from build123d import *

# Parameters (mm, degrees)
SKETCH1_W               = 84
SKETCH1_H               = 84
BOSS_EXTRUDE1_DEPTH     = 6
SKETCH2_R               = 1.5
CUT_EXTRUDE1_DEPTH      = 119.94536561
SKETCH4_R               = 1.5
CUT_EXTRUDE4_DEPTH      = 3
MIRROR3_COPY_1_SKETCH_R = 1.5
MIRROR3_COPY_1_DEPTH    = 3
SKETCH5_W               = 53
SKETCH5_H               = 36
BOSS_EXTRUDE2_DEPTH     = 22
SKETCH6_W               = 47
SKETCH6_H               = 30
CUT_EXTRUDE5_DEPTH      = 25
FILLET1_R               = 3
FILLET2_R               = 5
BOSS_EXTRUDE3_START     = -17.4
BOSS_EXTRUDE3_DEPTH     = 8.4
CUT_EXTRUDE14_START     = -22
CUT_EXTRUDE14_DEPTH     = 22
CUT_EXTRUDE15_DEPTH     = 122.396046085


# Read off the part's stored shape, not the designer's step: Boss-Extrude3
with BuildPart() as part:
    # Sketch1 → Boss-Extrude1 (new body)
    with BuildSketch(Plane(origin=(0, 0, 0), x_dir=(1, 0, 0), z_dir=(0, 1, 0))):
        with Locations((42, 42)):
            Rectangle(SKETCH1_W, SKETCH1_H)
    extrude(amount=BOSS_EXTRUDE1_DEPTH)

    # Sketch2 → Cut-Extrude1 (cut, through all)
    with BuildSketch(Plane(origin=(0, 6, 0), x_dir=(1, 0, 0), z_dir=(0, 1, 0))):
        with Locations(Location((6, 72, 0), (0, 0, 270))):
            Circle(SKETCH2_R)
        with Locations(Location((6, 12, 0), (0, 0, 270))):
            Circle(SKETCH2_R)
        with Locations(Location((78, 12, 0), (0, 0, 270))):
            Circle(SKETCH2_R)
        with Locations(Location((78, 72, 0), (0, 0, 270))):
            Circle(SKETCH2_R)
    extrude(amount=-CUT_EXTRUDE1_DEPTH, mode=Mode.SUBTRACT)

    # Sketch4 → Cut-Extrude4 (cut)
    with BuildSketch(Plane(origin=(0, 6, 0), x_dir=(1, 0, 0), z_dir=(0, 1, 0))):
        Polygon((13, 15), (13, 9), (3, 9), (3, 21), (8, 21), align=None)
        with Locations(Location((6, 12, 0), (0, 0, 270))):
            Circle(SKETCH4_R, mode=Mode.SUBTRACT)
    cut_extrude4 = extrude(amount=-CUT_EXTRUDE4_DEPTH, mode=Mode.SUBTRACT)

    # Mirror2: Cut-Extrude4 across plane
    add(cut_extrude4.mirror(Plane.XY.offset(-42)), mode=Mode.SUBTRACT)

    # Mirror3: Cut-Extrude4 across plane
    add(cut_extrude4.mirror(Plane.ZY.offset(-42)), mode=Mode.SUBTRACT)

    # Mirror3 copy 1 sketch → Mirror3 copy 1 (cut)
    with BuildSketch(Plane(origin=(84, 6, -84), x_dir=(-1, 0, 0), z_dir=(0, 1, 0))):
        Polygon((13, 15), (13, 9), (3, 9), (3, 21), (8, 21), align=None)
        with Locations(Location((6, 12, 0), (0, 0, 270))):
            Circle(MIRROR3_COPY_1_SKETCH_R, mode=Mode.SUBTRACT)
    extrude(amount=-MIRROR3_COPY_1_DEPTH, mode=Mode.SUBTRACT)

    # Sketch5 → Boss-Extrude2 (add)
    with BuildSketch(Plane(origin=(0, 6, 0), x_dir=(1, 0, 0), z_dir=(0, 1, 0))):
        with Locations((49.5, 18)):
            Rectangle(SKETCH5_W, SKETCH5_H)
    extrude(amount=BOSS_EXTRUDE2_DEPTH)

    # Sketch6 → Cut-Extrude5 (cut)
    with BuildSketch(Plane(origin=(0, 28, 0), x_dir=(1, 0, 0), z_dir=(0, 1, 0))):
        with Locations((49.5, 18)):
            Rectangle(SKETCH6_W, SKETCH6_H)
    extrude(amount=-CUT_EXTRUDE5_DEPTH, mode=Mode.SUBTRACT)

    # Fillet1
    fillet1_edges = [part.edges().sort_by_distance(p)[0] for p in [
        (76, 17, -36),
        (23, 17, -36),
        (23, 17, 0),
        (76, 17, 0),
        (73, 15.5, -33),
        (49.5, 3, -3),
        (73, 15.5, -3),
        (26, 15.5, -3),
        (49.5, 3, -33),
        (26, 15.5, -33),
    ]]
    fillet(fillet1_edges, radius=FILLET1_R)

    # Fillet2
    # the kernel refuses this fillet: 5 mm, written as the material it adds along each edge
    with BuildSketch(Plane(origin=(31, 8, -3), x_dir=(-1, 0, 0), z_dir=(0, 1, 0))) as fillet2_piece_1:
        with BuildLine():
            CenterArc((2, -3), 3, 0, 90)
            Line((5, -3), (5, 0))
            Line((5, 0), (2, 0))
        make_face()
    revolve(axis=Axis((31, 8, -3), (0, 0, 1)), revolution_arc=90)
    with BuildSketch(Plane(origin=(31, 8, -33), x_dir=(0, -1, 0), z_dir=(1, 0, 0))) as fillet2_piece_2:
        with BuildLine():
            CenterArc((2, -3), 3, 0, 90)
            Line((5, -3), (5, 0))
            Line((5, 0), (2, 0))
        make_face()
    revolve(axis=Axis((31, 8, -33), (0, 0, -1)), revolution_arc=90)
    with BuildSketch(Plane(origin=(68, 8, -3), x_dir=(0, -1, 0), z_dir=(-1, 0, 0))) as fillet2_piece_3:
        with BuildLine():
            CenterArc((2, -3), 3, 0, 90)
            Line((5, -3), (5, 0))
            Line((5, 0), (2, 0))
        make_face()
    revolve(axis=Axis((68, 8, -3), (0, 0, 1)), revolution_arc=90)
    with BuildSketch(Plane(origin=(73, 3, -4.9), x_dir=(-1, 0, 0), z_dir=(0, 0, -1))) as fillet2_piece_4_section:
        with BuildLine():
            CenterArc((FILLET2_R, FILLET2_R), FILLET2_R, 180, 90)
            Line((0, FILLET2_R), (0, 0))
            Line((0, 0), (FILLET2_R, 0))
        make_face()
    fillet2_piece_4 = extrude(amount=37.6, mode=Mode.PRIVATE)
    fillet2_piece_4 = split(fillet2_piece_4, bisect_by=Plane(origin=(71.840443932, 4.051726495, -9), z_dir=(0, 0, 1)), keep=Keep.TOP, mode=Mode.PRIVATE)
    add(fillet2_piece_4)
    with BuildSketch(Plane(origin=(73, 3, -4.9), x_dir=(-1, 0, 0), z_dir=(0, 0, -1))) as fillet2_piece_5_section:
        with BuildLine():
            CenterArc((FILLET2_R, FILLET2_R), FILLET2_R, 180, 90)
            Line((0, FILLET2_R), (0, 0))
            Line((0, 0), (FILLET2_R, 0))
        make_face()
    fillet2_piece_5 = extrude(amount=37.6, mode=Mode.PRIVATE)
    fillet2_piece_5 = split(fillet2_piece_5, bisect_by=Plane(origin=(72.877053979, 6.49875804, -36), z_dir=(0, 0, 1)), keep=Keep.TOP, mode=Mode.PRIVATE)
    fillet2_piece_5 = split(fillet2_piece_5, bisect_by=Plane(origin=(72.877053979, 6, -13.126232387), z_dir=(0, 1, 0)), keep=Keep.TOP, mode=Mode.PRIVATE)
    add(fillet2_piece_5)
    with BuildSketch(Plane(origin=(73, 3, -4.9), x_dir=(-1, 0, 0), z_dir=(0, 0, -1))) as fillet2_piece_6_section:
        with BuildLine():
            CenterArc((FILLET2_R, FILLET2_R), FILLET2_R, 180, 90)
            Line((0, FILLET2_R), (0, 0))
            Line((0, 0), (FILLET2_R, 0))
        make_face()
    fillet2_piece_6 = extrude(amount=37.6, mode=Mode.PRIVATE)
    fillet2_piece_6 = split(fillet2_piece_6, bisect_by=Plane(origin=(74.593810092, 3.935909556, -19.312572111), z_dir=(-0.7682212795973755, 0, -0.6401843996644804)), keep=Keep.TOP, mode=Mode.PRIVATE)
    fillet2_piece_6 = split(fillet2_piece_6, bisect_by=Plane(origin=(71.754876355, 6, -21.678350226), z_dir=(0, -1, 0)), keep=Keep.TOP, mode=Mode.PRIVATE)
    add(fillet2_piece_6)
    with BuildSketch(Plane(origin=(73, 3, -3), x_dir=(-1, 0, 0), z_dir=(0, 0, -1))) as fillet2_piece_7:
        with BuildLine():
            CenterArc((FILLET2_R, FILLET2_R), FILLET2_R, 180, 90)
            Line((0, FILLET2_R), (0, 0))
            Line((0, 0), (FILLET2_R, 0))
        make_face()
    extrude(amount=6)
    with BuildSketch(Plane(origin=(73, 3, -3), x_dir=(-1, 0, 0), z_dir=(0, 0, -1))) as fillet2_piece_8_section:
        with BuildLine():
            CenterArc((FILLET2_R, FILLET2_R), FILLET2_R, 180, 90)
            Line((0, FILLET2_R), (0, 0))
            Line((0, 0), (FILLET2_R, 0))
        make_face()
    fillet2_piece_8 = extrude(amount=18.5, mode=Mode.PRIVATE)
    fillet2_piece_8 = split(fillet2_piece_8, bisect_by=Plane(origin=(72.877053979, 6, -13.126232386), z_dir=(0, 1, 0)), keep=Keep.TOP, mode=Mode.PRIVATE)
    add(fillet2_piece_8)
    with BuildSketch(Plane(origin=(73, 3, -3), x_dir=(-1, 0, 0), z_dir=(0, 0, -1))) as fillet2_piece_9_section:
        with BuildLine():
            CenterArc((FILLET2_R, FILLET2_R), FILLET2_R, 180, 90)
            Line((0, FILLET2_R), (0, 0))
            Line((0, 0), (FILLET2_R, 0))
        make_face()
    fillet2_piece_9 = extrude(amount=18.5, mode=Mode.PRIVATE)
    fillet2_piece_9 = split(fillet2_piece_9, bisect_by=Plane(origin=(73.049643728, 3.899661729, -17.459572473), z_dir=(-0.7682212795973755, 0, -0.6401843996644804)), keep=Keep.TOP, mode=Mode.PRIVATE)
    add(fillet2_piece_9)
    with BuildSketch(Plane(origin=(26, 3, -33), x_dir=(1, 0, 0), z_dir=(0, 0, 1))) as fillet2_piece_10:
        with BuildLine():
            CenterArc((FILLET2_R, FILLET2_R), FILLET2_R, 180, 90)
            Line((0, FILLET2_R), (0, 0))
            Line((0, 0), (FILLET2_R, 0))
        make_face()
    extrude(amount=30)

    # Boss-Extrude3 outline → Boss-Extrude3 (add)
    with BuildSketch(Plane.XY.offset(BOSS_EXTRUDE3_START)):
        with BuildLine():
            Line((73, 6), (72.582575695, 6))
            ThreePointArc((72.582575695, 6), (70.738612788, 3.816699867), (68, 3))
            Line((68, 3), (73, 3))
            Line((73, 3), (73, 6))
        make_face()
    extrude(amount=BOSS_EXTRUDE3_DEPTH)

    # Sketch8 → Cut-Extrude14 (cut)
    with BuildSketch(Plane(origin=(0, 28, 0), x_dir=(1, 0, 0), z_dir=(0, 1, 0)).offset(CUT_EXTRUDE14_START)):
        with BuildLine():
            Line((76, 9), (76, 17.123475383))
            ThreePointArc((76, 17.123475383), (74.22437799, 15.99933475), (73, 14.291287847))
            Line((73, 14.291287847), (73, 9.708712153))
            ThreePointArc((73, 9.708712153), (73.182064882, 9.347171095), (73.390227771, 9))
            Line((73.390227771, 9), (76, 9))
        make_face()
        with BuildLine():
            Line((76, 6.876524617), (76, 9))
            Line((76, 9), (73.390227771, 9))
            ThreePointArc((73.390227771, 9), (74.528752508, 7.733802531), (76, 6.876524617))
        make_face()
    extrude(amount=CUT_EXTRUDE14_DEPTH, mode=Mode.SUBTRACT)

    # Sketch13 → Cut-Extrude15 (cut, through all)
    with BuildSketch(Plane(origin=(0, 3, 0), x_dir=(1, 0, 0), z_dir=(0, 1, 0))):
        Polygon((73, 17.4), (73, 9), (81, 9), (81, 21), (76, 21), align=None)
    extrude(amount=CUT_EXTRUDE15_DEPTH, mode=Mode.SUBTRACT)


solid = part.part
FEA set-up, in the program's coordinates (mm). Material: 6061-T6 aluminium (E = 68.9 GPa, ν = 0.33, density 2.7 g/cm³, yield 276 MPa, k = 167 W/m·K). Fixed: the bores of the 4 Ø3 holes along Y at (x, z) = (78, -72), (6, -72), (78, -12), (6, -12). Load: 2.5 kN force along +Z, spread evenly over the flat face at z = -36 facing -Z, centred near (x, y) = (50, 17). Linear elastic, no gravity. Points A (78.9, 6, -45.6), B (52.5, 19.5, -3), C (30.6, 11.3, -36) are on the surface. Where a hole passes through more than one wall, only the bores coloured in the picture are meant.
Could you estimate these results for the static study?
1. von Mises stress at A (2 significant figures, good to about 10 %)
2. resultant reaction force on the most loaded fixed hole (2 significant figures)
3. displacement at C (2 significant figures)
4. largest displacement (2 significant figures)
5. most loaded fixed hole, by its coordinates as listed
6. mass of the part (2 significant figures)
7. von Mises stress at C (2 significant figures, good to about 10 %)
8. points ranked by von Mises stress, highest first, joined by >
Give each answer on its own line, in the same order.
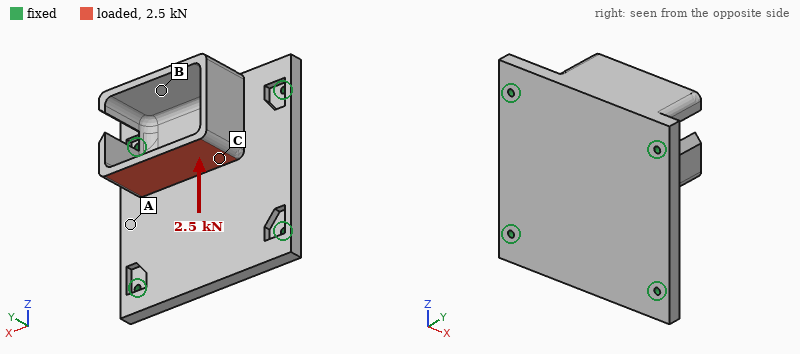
28 MPa
1.1 kN
0.045 mm
0.27 mm
(78, -72)
130 g
67 MPa
C > A > B
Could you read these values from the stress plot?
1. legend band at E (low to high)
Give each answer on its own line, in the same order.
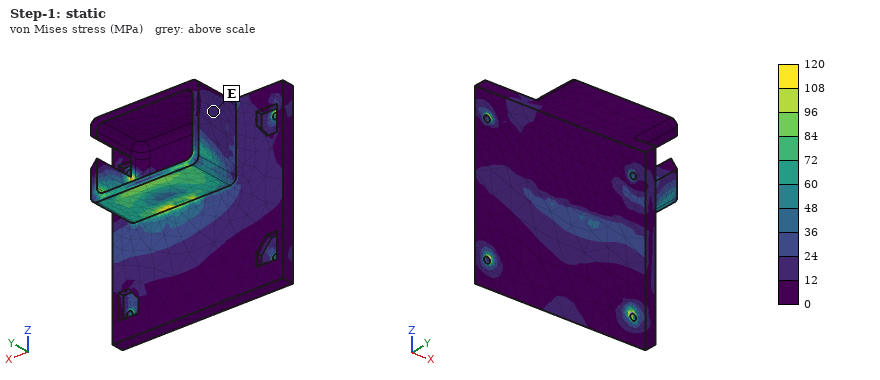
12 to 24 MPa
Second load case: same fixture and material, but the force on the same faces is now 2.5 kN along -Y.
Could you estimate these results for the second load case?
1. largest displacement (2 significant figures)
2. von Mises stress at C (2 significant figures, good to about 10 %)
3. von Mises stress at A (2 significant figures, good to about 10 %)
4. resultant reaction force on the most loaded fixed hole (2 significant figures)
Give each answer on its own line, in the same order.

0.14 mm
39 MPa
54 MPa
1.2 kN
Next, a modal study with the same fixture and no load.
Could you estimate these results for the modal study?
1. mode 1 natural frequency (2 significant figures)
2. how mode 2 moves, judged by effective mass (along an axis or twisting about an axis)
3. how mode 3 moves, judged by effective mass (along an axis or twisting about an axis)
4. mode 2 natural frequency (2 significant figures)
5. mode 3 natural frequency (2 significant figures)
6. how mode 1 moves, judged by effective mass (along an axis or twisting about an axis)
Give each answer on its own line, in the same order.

3200 Hz
along Y
twisting about X
3800 Hz
4800 Hz
along Y
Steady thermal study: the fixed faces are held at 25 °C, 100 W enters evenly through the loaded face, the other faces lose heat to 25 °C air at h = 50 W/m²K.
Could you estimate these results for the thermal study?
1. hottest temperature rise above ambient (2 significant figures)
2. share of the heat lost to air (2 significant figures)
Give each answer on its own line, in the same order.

71 K
24 %
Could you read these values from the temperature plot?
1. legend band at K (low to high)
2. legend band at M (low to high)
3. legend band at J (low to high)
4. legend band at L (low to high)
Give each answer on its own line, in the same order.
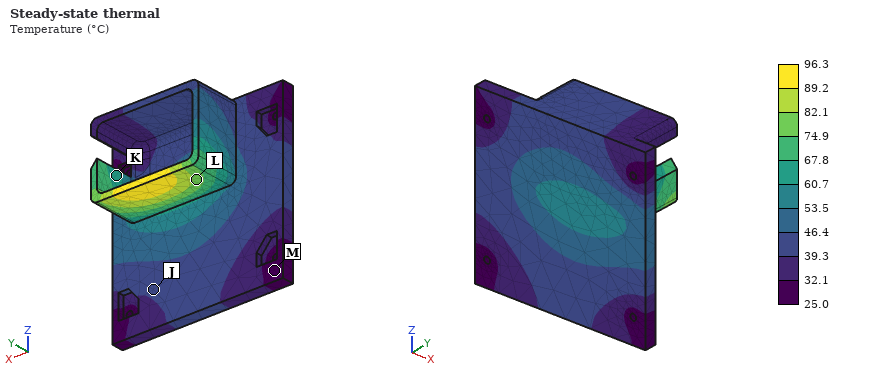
60.7 to 67.8 °C
25.0 to 32.1 °C
39.3 to 46.4 °C
74.9 to 82.1 °C
